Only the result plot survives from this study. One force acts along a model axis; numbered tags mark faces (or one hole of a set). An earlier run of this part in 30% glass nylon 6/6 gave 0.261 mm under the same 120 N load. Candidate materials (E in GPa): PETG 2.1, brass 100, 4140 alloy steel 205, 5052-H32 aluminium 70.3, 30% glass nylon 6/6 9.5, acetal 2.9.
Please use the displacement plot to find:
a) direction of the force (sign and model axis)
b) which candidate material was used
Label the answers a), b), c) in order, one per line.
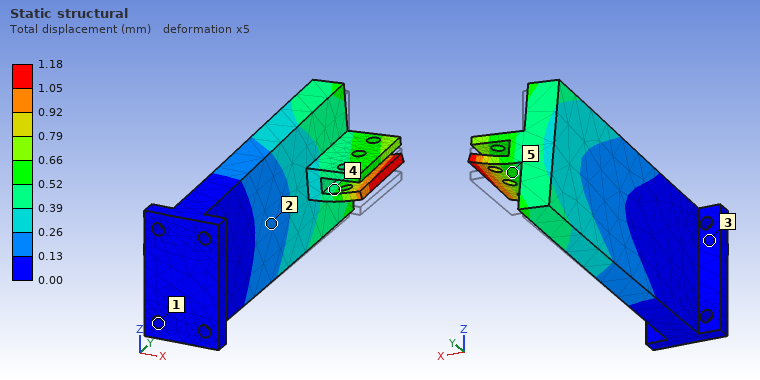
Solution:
a) +Z
b) PETG
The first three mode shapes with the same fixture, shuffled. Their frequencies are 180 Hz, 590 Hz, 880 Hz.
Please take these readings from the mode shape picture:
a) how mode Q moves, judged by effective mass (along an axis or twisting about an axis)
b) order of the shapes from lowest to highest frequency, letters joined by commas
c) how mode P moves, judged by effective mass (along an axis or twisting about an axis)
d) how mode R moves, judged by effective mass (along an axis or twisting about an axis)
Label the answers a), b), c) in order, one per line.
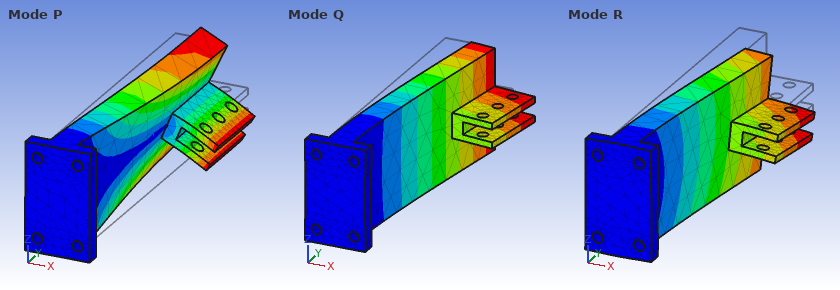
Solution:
a) along X
b) Q, R, P
c) twisting about Y
d) along Z
